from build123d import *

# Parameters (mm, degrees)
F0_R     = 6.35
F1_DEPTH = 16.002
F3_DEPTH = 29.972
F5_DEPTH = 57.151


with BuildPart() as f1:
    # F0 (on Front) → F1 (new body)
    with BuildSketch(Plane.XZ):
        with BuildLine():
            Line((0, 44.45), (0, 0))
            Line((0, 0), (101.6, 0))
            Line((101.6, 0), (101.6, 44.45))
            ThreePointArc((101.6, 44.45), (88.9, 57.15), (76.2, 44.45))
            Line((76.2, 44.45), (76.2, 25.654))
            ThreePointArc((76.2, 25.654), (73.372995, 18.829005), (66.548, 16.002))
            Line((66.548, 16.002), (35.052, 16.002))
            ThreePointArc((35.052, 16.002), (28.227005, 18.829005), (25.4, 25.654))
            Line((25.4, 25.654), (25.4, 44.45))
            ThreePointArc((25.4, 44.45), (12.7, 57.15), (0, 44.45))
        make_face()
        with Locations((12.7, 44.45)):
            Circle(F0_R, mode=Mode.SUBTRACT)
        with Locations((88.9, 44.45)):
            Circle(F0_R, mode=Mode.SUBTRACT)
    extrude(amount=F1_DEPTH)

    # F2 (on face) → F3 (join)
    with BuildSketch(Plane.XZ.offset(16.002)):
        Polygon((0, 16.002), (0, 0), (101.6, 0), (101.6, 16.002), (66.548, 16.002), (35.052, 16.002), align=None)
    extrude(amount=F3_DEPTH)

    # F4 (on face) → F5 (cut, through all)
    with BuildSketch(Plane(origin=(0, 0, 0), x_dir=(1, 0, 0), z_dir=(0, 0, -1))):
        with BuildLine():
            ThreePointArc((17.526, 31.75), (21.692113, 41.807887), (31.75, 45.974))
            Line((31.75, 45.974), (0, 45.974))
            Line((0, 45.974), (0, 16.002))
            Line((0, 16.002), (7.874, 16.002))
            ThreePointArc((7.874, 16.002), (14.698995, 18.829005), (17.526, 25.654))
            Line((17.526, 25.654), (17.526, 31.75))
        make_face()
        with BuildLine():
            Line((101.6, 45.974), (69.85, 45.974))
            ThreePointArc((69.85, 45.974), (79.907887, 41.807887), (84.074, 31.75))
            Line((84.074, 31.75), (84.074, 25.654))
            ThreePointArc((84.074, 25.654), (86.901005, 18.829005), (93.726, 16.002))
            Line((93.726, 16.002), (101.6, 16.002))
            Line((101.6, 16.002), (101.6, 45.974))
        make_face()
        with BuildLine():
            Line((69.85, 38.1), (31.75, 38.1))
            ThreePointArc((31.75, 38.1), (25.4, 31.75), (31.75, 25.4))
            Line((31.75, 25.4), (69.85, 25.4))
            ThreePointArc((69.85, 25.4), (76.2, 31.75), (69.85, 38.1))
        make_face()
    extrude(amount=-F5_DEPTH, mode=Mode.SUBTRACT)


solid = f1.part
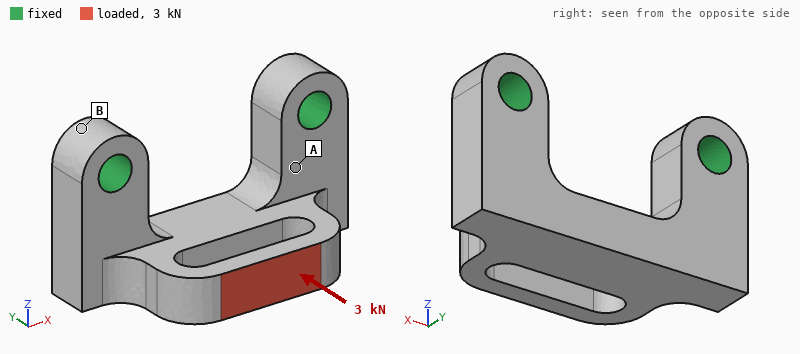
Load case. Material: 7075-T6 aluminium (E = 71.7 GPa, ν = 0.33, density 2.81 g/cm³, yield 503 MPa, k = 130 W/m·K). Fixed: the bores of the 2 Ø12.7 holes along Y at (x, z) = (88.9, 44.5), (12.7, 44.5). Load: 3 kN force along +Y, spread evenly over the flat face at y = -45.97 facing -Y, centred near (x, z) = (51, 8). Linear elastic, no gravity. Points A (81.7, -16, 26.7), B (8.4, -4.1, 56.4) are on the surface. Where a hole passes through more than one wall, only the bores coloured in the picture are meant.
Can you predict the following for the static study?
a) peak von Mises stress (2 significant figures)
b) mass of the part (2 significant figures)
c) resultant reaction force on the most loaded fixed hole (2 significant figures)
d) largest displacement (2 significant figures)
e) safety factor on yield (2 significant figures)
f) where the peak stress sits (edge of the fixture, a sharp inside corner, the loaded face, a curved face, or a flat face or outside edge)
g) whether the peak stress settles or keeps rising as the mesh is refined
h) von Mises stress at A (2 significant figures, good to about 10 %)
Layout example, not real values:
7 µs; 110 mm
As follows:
100 MPa; 210 g; 1.5 kN; 0.12 mm; 4.9; a curved face; settles; 26 MPa
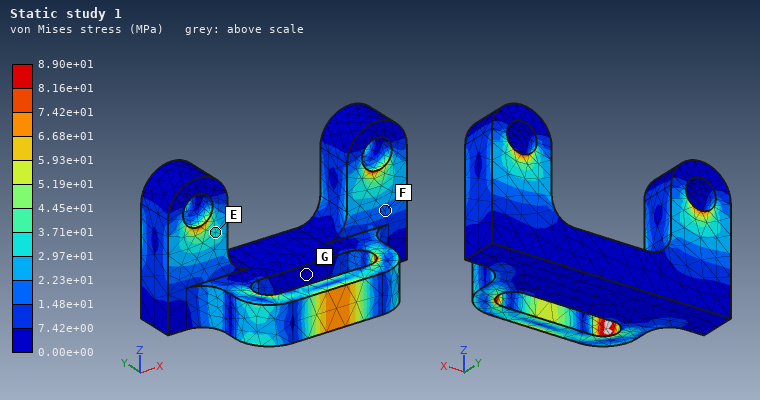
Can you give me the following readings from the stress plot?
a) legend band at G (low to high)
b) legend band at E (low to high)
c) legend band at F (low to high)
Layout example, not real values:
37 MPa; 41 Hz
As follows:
0.00e+00 to 7.42e+00 MPa; 2.97e+01 to 3.71e+01 MPa; 1.48e+01 to 2.23e+01 MPa
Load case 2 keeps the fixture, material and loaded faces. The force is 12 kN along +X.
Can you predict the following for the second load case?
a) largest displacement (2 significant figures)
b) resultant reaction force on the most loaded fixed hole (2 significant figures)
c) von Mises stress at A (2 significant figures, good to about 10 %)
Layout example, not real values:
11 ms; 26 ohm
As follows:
0.27 mm; 8.4 kN; 74 MPa
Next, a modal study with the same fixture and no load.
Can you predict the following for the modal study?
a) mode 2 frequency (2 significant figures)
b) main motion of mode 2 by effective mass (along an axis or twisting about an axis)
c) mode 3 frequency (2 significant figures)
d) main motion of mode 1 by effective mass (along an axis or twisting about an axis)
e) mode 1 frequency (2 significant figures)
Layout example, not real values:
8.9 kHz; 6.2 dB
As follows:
5500 Hz; along X; 6700 Hz; along Y; 3100 Hz
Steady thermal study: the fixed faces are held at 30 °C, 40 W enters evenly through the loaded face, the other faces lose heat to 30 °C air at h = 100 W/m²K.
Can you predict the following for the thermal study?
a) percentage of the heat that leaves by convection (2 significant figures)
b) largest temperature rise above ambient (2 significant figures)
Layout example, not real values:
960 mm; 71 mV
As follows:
41 %; 45 K
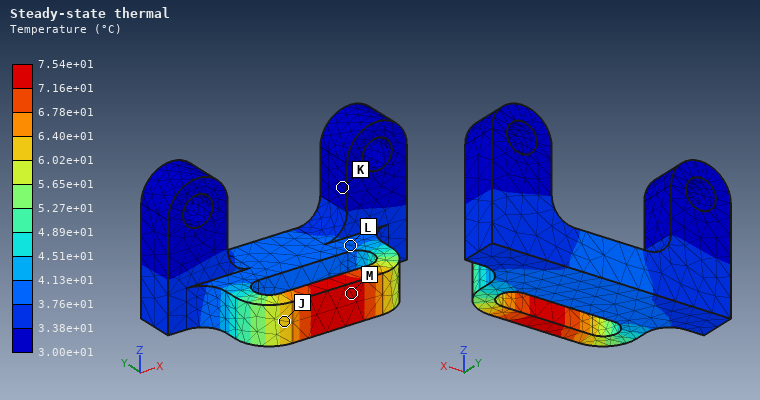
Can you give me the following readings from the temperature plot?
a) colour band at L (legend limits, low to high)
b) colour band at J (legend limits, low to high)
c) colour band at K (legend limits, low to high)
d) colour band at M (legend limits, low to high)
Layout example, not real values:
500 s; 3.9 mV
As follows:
3.76e+01 to 4.13e+01 °C; 6.02e+01 to 6.40e+01 °C; 3.00e+01 to 3.38e+01 °C; 7.16e+01 to 7.54e+01 °C
